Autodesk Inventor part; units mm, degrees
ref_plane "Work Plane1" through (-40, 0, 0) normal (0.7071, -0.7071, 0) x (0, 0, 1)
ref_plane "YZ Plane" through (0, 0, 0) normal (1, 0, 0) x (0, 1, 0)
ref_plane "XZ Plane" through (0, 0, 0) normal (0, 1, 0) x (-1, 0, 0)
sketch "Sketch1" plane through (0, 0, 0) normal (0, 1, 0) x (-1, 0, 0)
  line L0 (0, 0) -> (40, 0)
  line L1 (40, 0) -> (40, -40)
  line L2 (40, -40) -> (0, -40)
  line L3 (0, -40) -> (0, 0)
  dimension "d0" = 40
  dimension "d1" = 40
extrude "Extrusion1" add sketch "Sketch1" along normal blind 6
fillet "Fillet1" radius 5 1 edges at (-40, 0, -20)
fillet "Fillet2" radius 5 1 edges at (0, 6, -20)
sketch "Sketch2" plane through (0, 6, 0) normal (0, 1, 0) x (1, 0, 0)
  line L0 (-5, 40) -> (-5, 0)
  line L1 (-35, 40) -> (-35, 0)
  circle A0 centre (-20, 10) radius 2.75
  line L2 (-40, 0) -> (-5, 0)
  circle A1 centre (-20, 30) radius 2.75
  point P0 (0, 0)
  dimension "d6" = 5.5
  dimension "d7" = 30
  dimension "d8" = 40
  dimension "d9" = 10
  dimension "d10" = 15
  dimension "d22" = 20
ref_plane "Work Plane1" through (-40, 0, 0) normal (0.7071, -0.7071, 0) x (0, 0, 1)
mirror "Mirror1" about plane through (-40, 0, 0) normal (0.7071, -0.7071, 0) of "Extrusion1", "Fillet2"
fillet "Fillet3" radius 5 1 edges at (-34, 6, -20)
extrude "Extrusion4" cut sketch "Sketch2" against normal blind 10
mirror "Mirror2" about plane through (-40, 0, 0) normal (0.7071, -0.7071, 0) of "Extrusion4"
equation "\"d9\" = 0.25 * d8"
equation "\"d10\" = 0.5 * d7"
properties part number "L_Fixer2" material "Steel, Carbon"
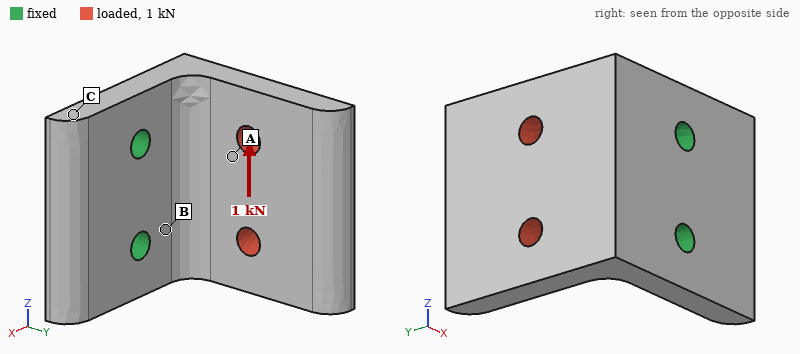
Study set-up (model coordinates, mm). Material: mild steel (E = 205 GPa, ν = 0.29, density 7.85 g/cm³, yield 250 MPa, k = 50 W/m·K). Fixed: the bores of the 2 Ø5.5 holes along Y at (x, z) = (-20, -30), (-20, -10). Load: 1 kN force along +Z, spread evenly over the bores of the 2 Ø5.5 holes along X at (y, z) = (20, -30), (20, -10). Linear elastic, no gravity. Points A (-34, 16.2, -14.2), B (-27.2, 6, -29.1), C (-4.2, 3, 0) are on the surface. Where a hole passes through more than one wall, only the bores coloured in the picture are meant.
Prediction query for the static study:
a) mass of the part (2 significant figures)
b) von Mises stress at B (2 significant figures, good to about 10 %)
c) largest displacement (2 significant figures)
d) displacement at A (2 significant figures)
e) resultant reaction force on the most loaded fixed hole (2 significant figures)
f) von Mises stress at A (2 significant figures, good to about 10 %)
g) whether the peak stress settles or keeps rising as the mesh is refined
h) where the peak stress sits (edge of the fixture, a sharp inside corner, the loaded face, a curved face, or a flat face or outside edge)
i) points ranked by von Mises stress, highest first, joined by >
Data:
130 g
32 MPa
19 µm
7.6 µm
1.1 kN
15 MPa
keeps rising
edge of the fixture
B > A > C
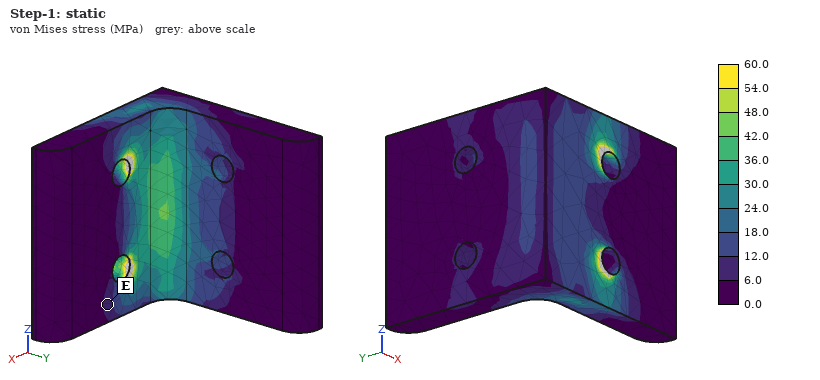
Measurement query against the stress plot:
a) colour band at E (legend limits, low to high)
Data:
6.0 to 12.0 MPa
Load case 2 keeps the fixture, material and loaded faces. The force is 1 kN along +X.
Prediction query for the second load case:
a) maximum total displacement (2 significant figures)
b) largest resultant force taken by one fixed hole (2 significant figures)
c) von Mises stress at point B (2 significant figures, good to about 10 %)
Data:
75 µm
510 N
79 MPa
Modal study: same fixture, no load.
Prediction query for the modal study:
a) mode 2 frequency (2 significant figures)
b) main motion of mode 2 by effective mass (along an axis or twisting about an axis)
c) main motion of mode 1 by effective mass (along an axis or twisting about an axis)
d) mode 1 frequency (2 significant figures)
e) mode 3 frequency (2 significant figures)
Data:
4800 Hz
along Z
along X
2500 Hz
8000 Hz
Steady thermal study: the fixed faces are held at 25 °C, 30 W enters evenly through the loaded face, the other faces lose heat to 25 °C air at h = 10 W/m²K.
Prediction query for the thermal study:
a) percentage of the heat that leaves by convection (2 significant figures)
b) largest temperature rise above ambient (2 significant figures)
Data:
7.9 %
76 K
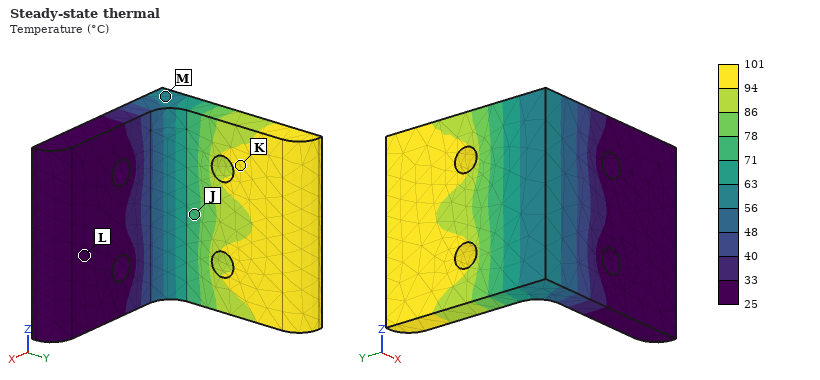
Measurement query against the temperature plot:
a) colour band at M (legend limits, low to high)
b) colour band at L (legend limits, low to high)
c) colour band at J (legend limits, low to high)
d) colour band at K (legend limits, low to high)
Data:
56 to 63 °C
25 to 33 °C
71 to 78 °C
94 to 101 °C
